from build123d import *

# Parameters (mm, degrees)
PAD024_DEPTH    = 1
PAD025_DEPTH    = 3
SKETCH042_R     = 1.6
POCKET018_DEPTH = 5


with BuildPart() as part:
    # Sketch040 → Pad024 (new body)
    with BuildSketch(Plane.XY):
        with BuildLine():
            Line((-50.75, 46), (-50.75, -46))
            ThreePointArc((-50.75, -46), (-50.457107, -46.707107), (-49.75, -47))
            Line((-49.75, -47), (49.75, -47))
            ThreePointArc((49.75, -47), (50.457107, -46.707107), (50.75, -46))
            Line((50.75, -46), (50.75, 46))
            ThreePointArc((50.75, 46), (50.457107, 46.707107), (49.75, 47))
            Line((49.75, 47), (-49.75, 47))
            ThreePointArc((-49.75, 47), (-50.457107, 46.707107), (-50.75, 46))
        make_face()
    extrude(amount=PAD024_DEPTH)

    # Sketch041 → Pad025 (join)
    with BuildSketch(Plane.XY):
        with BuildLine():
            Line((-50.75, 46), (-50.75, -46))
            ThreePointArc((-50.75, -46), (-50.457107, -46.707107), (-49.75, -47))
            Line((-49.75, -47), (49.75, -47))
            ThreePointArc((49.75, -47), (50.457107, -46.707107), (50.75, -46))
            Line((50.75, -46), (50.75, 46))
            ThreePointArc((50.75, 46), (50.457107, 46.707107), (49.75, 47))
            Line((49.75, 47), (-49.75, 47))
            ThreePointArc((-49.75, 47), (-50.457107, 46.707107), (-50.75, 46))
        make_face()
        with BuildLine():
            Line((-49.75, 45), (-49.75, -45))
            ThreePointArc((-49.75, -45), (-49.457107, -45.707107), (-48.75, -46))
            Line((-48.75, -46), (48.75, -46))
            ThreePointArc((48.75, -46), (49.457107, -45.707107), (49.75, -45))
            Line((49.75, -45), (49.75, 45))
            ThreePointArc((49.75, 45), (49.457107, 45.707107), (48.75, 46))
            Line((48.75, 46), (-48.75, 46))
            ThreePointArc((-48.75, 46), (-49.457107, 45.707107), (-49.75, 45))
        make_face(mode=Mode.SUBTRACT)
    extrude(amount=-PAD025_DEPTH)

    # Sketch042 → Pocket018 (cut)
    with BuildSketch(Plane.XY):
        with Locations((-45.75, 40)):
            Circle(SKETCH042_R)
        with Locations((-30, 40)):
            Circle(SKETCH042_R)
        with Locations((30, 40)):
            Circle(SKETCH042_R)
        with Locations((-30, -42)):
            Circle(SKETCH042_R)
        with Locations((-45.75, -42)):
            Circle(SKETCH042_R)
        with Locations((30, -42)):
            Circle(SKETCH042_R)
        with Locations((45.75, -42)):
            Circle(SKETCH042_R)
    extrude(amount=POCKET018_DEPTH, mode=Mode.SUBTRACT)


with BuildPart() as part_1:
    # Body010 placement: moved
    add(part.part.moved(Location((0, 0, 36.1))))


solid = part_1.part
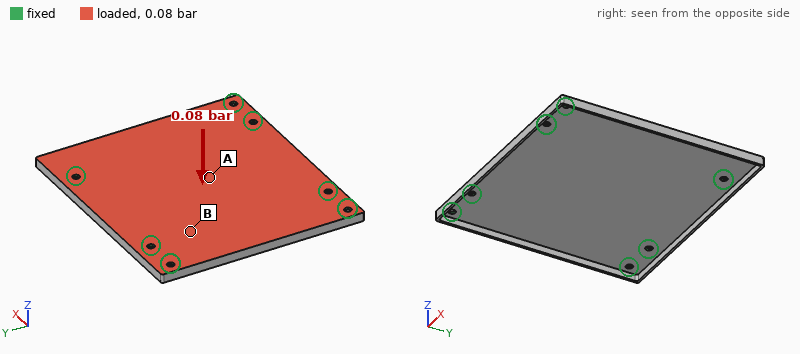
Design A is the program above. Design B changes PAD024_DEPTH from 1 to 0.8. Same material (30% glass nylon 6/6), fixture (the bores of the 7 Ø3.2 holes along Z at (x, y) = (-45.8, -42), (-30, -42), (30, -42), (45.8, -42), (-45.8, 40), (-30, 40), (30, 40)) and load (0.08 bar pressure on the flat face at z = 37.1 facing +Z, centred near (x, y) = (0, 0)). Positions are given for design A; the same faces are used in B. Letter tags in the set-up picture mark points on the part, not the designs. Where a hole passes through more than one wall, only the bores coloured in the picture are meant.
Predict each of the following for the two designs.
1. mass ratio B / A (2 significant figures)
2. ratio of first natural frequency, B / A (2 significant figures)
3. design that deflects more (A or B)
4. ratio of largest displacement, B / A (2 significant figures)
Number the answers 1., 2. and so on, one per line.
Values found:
1. 0.82
2. 0.82
3. B
4. 1.9
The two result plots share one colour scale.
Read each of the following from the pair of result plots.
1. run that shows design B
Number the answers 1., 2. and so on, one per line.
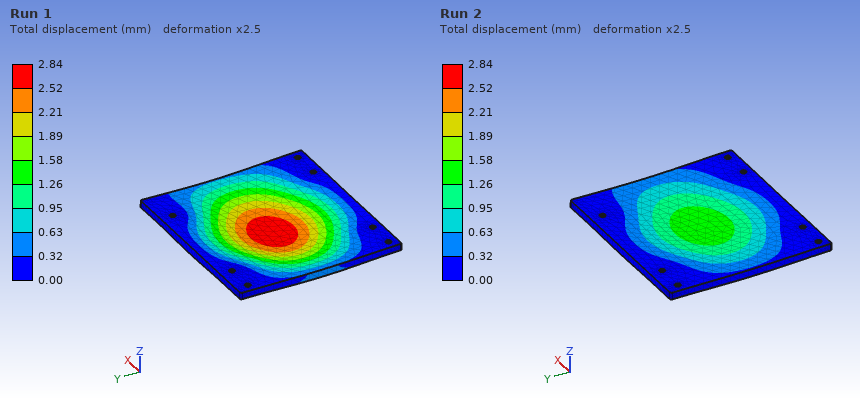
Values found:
1. Run 1
